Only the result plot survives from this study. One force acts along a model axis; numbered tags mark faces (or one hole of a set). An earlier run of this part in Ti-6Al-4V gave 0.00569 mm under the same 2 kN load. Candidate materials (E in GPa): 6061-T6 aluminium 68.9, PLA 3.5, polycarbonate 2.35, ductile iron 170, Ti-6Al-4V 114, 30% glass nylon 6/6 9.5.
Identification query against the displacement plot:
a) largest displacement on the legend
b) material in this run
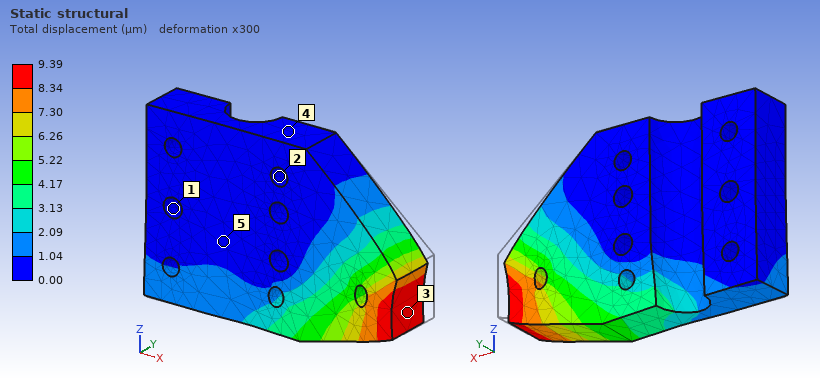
9.39 µm
6061-T6 aluminium
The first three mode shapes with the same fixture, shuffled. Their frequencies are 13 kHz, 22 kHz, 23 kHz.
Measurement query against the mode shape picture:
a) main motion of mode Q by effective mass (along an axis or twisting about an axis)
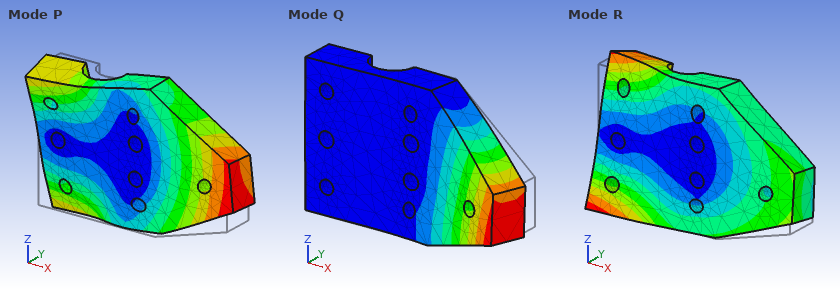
along Y
